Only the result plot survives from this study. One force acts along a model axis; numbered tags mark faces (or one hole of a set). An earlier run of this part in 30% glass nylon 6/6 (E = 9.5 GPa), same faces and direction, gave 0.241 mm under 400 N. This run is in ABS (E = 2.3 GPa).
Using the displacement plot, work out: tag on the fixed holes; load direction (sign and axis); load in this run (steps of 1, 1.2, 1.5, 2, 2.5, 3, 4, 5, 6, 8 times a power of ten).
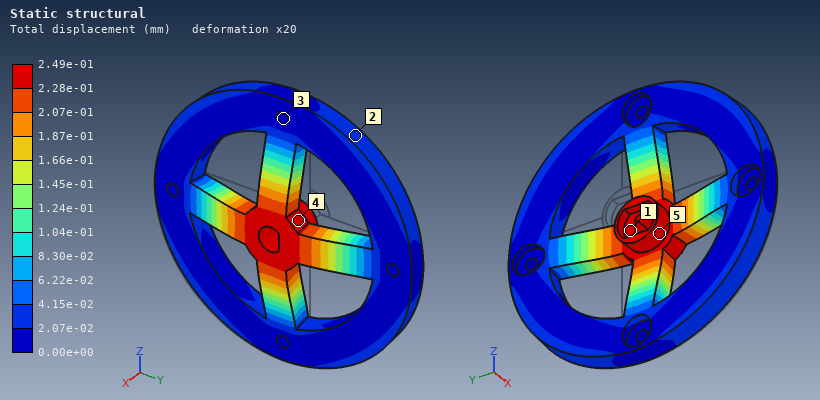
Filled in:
3
+X
100 N
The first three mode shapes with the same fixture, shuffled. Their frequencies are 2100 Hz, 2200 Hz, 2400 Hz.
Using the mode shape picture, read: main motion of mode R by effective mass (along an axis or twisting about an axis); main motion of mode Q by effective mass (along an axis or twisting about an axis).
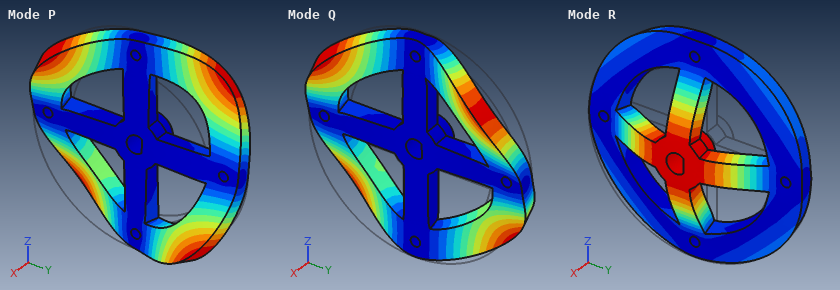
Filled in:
along X
twisting about Y
